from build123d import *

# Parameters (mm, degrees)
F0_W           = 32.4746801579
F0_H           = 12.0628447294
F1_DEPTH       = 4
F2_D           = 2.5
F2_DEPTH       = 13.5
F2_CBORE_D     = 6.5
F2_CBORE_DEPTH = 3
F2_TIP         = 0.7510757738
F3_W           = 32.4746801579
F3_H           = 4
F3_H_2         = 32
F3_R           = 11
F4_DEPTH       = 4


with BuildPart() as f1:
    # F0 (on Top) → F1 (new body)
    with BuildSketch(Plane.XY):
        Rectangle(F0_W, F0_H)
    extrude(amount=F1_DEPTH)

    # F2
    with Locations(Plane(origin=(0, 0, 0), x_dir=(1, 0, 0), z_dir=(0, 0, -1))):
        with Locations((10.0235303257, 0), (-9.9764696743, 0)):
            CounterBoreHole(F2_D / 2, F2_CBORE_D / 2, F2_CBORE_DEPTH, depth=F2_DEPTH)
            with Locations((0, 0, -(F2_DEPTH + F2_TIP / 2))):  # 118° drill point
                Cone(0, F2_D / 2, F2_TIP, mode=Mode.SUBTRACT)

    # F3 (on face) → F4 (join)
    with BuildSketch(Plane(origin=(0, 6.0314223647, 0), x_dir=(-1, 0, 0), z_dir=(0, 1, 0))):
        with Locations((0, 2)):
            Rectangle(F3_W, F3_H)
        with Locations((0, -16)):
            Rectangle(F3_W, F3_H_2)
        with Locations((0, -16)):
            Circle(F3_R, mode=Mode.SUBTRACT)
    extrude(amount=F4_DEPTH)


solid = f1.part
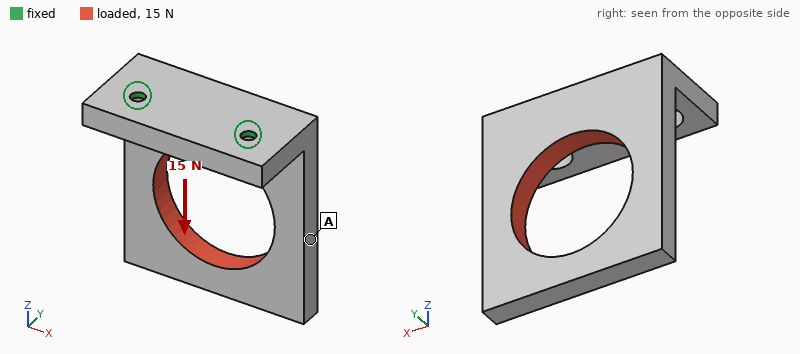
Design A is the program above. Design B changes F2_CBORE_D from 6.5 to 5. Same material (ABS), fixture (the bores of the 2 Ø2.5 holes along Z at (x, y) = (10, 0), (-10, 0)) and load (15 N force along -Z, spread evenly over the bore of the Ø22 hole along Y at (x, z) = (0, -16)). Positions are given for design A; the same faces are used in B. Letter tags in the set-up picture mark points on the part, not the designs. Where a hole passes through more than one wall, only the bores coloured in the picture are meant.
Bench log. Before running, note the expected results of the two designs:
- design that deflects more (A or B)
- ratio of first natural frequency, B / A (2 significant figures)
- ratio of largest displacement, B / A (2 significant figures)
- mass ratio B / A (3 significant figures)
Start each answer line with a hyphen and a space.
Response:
- A
- 1.1
- 0.81
- 1.02
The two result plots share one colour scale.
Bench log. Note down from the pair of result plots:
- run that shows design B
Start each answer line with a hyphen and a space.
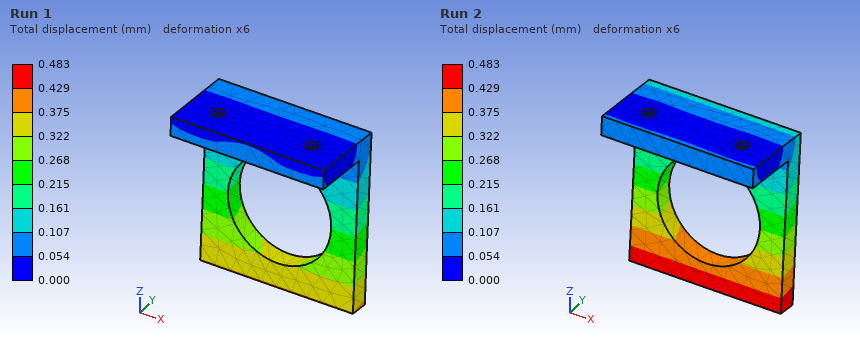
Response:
- Run 1
